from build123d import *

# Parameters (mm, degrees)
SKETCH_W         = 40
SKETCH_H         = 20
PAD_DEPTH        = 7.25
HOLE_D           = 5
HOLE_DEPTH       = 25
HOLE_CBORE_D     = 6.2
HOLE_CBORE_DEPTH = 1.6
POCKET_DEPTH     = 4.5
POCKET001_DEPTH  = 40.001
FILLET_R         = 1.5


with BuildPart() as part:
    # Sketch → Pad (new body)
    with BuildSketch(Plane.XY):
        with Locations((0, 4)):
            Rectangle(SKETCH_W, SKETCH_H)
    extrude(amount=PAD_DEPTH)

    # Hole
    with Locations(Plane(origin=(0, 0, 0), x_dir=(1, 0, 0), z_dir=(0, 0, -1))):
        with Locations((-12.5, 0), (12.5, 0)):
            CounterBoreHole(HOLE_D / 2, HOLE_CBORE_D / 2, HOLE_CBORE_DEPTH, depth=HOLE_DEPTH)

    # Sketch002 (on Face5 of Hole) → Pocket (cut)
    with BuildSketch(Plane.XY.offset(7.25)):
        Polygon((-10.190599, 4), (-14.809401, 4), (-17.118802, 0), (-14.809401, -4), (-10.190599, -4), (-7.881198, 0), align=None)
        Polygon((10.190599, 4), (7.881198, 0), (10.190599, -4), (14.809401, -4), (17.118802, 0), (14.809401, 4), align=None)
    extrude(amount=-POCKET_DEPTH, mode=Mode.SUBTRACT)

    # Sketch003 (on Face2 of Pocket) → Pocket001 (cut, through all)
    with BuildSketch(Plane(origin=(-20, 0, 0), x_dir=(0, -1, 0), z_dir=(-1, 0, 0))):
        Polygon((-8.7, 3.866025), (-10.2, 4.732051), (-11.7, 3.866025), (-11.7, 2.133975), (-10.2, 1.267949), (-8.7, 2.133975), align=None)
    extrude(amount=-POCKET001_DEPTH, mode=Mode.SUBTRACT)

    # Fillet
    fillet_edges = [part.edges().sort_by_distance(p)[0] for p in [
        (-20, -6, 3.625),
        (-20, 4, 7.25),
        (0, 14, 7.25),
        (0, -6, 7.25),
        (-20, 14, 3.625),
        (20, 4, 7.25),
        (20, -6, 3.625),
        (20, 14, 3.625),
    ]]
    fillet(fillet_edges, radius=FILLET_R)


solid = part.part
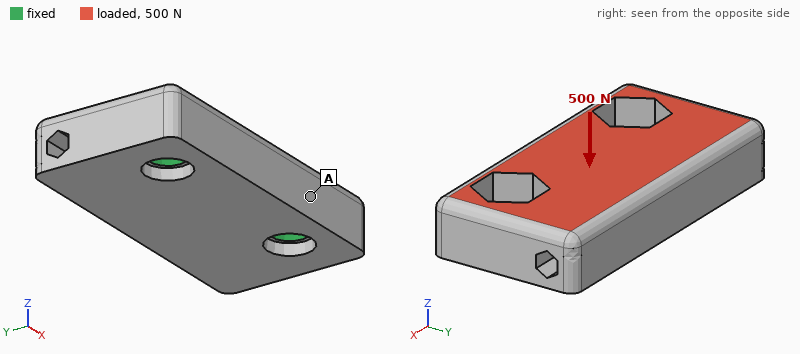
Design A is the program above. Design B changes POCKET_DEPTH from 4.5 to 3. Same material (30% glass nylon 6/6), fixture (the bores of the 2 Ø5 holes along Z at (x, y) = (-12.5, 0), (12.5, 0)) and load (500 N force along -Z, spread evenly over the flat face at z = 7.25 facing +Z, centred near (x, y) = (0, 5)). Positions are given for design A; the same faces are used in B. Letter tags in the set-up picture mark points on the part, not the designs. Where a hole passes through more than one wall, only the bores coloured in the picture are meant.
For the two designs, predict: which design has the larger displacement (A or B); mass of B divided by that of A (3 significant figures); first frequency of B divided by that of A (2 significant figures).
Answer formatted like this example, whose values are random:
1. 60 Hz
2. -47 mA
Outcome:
1. A
2. 1.02
3. 1.6
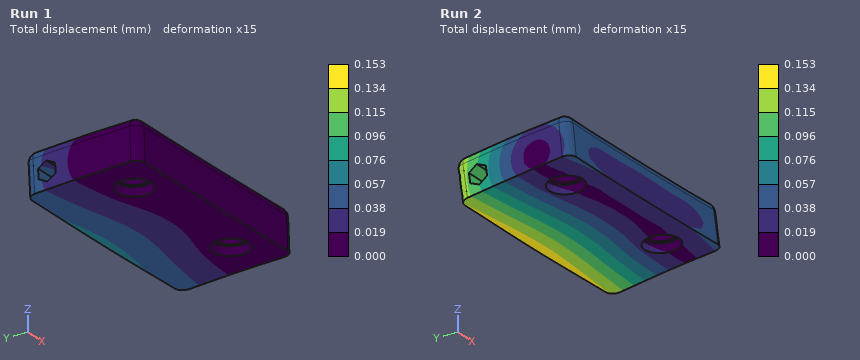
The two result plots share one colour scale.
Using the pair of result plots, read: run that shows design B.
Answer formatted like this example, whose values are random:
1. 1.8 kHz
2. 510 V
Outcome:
1. Run 1
